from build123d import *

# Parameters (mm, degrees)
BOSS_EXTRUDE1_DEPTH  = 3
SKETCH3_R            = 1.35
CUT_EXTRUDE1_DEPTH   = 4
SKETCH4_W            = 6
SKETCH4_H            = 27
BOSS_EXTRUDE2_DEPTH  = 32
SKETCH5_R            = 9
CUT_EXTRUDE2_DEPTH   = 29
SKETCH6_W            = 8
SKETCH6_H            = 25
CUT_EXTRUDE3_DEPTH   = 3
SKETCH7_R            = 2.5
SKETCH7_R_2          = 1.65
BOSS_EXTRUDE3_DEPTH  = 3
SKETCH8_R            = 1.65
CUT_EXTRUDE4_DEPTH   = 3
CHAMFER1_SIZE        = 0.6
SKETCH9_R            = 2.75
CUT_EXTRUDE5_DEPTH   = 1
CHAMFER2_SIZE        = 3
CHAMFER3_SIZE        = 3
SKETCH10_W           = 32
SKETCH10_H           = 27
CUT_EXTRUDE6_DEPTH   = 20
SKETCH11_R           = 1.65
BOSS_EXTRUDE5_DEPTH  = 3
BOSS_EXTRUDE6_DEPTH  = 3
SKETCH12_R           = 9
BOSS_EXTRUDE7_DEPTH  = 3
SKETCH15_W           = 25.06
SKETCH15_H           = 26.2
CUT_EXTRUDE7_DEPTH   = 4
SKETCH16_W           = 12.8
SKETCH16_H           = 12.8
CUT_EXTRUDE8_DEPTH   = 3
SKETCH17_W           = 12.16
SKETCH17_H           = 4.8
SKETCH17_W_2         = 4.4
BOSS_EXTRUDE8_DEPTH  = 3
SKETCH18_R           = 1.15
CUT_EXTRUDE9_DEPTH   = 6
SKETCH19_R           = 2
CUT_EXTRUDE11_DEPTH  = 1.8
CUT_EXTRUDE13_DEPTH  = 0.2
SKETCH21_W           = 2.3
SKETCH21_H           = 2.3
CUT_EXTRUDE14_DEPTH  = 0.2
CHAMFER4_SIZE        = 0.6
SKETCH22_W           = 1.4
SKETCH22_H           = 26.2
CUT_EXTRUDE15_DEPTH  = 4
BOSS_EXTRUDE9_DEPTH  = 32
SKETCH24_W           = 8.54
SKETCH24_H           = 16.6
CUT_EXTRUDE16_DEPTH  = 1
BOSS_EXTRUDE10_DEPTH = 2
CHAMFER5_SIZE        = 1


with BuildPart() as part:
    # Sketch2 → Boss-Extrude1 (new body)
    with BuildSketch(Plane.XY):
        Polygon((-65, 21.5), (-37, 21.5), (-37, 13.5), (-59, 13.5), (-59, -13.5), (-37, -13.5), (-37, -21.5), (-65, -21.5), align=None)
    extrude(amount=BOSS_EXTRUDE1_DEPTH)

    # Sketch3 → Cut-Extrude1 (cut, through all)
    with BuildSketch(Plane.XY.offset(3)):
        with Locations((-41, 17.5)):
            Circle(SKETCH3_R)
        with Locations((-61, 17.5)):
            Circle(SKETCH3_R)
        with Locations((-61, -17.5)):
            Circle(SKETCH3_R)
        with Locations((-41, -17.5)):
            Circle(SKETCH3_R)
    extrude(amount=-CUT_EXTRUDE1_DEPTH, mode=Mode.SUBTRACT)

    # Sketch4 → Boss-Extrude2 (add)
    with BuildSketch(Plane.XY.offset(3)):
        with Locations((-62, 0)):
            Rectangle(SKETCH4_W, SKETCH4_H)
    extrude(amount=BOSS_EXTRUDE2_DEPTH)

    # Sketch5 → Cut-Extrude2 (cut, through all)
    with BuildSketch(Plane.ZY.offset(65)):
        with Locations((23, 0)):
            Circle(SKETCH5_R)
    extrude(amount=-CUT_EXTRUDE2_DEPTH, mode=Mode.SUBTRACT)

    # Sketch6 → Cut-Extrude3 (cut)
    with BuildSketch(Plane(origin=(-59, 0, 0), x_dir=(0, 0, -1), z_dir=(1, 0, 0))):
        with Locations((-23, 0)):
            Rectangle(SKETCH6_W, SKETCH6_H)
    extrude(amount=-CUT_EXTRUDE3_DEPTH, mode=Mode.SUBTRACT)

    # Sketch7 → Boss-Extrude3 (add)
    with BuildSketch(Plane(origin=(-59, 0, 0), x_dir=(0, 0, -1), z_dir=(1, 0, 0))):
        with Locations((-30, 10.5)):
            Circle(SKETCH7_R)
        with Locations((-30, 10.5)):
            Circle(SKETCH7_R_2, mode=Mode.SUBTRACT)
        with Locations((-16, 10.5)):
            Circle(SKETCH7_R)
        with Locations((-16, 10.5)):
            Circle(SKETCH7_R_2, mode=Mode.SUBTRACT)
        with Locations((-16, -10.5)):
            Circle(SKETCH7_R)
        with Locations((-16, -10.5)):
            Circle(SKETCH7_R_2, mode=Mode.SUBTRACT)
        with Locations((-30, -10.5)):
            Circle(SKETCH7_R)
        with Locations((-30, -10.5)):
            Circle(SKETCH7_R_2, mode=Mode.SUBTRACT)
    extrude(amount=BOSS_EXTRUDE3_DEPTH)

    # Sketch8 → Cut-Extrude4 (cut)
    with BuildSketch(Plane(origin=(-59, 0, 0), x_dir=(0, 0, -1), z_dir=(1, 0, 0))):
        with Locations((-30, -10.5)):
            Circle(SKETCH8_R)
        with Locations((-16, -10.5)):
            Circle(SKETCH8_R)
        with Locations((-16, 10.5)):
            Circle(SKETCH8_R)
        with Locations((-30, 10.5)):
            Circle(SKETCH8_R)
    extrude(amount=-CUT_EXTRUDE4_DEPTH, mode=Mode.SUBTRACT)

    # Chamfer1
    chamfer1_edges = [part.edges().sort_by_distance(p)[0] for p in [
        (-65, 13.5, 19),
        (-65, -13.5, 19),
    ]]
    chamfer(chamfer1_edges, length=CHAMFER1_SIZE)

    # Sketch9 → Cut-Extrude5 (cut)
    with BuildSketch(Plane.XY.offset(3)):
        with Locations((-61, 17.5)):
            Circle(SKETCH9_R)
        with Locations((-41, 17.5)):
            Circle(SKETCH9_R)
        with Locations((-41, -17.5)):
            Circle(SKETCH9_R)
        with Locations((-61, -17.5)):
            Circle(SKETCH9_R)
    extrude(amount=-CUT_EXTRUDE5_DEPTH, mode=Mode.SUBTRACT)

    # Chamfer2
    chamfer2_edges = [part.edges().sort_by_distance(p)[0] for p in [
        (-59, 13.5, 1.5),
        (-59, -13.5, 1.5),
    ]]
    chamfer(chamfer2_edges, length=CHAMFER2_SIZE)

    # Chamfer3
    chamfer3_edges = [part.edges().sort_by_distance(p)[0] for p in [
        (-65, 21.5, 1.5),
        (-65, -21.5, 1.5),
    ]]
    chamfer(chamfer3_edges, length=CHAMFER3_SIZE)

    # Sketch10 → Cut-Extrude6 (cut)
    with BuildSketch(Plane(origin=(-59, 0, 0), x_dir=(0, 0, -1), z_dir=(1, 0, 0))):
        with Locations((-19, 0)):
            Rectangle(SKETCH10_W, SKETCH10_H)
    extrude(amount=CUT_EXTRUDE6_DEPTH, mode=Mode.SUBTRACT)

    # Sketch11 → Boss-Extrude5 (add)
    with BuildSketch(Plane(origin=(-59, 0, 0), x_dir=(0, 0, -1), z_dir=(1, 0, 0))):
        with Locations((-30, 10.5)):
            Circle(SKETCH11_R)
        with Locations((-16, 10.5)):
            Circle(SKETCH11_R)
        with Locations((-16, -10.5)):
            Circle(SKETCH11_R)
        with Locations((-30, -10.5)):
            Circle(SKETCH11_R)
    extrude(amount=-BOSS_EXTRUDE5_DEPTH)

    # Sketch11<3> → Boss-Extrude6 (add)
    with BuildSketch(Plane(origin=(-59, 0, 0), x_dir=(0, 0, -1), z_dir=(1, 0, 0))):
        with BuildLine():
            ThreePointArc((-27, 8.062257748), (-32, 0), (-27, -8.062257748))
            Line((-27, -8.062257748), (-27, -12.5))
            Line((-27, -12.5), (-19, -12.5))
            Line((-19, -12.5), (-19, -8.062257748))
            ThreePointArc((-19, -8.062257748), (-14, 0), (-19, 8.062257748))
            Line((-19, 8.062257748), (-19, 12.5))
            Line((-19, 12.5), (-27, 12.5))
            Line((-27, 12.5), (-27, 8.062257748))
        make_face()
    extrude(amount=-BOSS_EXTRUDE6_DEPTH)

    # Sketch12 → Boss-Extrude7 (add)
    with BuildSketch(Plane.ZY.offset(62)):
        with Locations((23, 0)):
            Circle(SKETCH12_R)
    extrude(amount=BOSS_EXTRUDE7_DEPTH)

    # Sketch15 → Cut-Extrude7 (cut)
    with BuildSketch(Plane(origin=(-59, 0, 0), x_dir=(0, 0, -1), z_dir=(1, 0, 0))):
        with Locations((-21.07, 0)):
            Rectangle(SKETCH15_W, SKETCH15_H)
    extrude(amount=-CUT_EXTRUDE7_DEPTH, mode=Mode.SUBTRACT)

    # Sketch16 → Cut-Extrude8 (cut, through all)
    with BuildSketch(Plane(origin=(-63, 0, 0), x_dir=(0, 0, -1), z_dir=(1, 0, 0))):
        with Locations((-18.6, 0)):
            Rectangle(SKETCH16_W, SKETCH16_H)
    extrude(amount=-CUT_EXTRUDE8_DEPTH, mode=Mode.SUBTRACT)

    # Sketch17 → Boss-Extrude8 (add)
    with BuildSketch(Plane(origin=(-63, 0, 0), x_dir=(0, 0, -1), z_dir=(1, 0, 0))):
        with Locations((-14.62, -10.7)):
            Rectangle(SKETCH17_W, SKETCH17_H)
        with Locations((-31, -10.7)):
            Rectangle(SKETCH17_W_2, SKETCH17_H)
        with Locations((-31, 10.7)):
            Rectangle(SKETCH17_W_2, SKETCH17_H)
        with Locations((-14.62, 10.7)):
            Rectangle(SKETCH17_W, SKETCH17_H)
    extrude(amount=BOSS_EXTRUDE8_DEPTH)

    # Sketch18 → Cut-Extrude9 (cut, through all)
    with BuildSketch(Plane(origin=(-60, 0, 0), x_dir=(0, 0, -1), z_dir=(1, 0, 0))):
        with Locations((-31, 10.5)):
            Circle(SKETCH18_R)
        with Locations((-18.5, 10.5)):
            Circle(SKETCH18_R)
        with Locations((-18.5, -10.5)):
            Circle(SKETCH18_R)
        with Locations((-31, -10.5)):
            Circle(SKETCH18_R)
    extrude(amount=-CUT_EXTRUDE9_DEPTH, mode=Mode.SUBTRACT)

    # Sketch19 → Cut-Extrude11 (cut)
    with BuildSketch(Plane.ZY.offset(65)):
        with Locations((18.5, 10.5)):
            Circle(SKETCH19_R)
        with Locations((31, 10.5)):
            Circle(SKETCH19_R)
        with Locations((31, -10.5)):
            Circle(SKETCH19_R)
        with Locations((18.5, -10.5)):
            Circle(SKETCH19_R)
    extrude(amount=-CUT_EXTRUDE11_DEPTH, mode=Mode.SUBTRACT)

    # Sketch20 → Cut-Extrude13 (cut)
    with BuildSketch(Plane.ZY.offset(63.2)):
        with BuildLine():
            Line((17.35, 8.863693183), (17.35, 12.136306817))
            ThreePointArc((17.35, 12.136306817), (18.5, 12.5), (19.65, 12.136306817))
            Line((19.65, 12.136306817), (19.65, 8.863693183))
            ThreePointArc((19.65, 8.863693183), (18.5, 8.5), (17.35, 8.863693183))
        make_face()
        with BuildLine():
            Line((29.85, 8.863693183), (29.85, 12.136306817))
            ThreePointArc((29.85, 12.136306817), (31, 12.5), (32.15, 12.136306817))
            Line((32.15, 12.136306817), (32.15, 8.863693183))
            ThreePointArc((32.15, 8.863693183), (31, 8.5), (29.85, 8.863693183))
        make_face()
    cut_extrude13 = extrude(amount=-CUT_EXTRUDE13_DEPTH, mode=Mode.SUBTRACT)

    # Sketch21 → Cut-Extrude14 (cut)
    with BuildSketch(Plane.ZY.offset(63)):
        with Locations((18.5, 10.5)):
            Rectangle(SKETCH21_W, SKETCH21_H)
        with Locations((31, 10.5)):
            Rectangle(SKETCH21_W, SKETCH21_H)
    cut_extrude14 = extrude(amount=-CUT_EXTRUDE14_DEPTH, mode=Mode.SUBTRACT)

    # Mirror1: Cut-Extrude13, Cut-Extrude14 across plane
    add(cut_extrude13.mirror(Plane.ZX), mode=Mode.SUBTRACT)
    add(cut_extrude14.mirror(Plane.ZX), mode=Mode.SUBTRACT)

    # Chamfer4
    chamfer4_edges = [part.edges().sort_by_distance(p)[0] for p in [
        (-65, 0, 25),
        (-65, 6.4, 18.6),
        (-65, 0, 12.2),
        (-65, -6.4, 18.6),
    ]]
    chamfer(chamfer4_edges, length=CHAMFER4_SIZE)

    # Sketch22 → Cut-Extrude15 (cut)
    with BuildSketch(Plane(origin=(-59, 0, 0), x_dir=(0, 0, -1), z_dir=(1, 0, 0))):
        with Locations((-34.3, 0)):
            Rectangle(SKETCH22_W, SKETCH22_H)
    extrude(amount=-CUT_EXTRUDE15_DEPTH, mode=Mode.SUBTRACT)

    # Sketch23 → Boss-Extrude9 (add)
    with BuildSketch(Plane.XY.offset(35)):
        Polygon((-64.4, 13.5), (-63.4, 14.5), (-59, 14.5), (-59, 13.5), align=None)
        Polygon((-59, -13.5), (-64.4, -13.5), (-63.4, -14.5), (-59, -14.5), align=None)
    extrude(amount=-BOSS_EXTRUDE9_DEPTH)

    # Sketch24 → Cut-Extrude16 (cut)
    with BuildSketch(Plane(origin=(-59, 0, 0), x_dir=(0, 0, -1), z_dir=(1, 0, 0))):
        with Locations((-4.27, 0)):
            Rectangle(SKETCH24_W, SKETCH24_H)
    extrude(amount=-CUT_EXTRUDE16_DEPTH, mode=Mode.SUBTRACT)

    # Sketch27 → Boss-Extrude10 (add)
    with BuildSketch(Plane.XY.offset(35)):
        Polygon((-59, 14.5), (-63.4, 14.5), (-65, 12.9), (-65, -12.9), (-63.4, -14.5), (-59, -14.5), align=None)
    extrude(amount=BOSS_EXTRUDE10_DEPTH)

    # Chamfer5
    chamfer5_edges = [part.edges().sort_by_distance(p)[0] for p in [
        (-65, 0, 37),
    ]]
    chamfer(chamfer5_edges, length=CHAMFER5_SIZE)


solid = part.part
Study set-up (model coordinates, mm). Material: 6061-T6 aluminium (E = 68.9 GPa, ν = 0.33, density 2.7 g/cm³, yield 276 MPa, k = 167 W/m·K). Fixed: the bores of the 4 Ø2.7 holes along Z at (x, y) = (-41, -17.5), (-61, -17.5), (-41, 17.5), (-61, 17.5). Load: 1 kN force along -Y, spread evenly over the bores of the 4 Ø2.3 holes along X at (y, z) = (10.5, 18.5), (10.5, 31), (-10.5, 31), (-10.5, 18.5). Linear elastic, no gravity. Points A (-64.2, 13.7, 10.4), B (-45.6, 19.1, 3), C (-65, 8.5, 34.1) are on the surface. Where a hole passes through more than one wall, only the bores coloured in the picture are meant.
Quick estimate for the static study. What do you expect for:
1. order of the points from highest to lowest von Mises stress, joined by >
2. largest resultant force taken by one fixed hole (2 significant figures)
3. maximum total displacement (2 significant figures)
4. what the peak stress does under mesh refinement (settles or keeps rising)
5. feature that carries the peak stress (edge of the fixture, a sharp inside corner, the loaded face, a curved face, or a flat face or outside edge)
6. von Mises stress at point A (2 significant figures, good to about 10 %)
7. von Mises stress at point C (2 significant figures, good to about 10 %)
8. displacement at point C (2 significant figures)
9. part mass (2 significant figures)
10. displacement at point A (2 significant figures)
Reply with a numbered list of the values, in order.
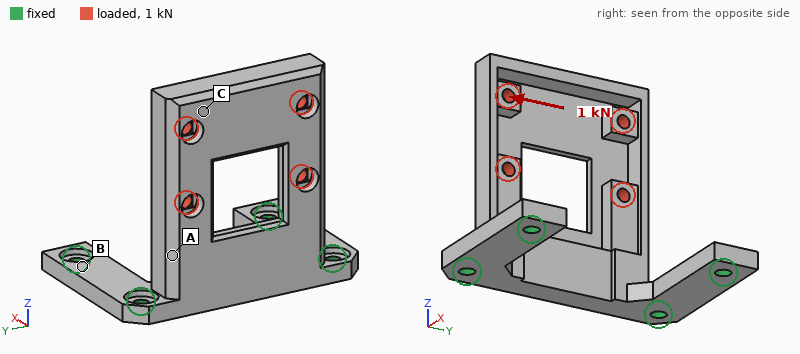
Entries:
1. A > C > B
2. 910 N
3. 0.23 mm
4. keeps rising
5. edge of the fixture
6. 110 MPa
7. 30 MPa
8. 0.13 mm
9. 12 g
10. 0.039 mm
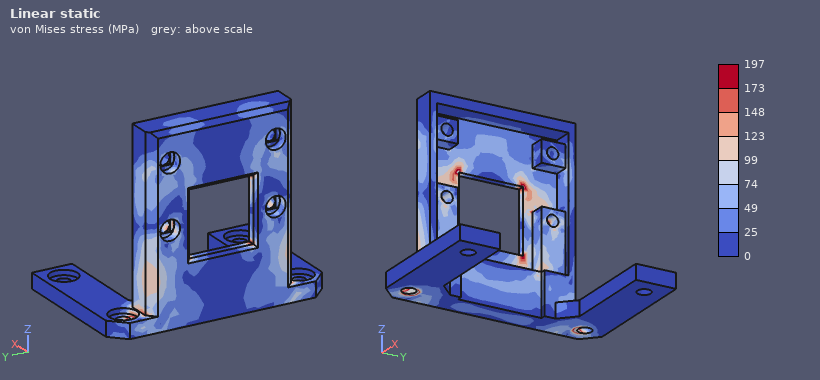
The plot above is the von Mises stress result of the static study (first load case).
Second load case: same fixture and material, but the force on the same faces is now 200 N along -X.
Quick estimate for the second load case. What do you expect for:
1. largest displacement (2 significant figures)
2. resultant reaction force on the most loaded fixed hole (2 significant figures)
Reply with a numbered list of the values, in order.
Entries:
1. 0.35 mm
2. 130 N
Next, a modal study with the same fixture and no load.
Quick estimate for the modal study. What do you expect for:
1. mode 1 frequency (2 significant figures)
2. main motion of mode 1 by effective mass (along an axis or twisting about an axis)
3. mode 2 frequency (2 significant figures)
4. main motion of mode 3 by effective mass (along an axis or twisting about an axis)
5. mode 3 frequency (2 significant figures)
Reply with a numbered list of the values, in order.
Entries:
1. 1900 Hz
2. along X
3. 4500 Hz
4. along Y
5. 8100 Hz
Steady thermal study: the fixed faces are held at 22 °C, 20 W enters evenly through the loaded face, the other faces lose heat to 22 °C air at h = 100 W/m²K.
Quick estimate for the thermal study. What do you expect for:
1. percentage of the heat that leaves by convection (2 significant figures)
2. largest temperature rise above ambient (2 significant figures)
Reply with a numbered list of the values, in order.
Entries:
1. 39 %
2. 40 K
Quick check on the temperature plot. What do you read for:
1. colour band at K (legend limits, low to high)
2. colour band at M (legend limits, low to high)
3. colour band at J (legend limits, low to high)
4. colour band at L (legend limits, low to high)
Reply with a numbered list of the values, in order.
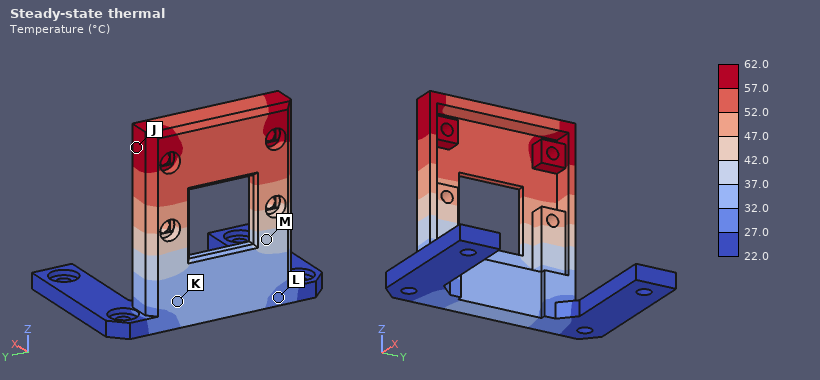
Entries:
1. 32.0 to 37.0 °C
2. 37.0 to 42.0 °C
3. 57.0 to 62.0 °C
4. 27.0 to 32.0 °C
